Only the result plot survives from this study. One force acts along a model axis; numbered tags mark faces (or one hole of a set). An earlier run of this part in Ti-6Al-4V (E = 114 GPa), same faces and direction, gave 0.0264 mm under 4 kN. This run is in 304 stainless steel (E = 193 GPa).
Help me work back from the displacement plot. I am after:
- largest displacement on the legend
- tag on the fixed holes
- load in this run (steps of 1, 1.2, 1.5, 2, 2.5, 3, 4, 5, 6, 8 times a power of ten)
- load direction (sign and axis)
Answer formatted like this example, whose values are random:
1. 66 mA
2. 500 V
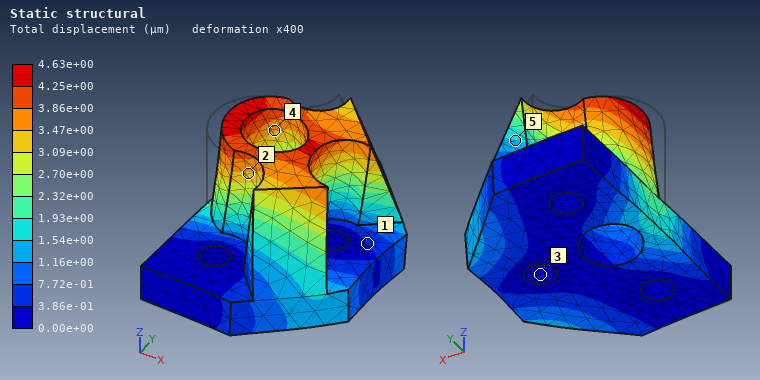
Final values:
1. 4.63e+00 µm
2. 3
3. 1.2 kN
4. +X
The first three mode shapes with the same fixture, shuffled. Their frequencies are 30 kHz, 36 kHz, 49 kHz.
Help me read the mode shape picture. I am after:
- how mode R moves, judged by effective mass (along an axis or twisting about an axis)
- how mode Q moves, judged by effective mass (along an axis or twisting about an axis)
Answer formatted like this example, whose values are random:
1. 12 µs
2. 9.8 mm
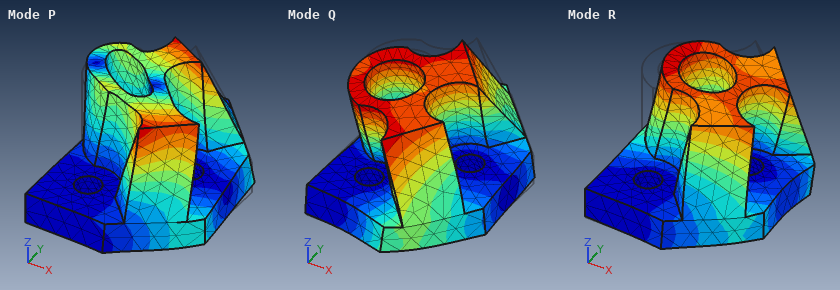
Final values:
1. along X
2. along Y
